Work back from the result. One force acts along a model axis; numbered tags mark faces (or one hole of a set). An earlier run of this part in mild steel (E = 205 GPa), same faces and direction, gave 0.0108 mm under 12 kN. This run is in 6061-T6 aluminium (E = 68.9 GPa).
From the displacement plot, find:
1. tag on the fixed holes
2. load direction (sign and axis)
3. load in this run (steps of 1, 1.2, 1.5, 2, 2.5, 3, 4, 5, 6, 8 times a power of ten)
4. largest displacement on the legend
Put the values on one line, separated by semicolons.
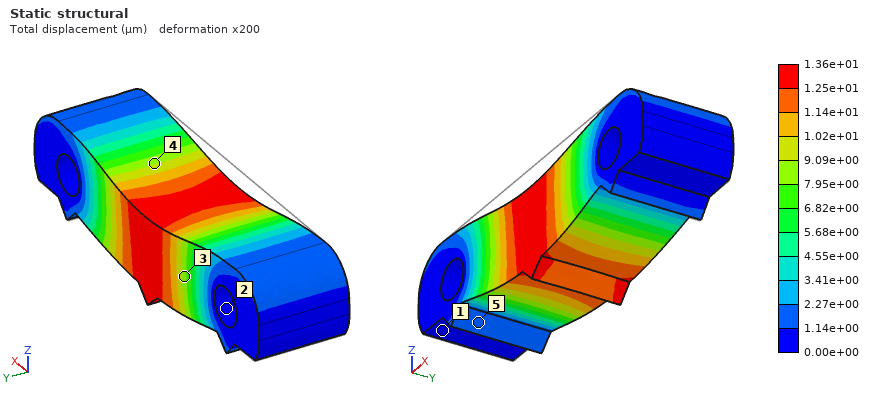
2; -Z; 5 kN; 1.36e+01 µm
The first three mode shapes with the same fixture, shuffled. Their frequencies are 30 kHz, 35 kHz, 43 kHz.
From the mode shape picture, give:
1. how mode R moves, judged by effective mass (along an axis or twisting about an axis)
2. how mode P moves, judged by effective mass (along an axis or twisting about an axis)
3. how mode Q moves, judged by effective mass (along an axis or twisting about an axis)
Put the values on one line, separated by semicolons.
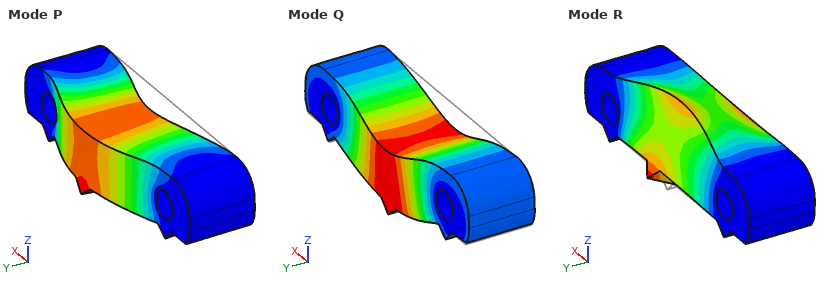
twisting about X; along Y; along Z
